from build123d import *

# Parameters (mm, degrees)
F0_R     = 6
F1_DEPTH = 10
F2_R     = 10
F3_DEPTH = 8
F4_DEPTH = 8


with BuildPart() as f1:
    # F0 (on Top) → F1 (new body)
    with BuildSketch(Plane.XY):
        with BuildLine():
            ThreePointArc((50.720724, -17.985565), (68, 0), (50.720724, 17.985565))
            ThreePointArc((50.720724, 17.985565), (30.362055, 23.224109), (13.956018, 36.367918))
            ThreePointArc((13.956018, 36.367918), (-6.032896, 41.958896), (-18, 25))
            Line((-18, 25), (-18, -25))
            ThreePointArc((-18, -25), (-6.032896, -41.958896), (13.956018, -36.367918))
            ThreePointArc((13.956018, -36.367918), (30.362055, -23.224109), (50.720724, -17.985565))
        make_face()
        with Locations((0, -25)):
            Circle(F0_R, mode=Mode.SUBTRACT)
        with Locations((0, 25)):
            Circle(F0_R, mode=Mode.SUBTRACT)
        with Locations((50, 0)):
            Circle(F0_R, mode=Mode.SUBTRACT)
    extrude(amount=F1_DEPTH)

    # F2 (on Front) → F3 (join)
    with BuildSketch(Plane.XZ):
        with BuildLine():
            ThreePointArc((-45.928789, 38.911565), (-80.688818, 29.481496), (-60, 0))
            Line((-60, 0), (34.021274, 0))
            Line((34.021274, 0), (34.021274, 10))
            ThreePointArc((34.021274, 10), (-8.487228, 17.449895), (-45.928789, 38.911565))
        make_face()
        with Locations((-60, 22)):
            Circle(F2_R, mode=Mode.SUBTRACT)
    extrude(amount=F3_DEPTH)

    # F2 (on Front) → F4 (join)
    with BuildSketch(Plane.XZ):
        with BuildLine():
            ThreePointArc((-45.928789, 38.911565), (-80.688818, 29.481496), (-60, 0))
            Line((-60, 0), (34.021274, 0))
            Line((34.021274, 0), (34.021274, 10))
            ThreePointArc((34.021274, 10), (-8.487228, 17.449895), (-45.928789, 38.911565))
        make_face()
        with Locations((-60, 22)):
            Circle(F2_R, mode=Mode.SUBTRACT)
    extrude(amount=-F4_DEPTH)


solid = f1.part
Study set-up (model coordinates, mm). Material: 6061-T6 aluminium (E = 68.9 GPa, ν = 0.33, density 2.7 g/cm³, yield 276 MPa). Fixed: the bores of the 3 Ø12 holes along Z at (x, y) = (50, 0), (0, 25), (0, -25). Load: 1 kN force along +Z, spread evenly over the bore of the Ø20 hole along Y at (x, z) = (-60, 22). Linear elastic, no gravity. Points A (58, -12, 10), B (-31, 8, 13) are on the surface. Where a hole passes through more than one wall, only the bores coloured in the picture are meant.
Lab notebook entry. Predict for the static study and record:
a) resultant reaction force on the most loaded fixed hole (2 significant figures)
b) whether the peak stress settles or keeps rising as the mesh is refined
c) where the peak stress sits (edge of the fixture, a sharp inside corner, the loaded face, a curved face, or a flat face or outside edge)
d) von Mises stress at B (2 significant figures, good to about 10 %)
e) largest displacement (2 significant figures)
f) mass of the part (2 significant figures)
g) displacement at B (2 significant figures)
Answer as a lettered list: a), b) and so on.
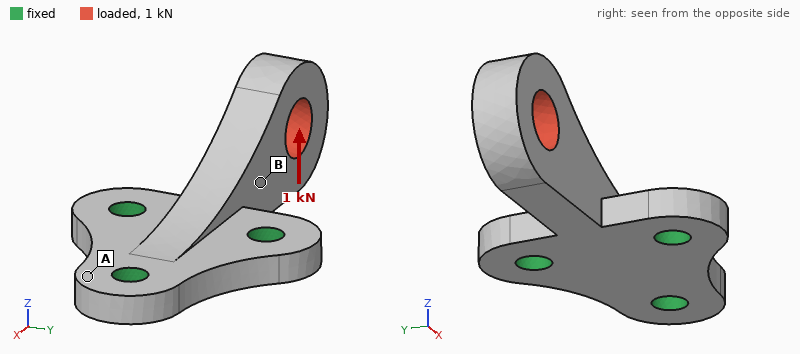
a) 970 N
b) keeps rising
c) edge of the fixture
d) 10 MPa
e) 0.22 mm
f) 210 g
g) 0.067 mm
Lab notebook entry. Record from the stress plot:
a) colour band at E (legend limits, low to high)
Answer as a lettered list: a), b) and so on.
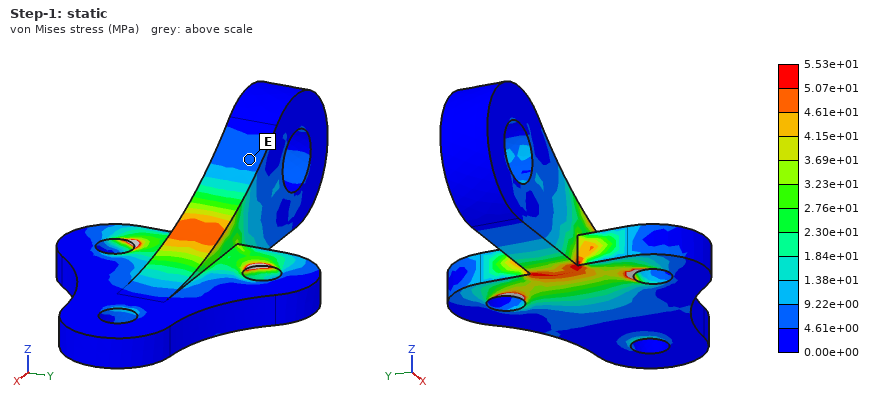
a) 4.61e+00 to 9.22e+00 MPa
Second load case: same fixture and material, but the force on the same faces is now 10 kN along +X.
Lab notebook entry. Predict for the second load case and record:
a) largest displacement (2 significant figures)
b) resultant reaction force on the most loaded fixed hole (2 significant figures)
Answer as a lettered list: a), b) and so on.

a) 0.63 mm
b) 3.5 kN
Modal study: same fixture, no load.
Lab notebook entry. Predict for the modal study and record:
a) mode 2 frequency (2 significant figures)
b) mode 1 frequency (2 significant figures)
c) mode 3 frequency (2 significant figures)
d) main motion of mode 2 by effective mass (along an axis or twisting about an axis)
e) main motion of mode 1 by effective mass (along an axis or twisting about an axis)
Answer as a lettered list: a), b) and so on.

a) 2000 Hz
b) 1600 Hz
c) 5300 Hz
d) along Y
e) along Z
